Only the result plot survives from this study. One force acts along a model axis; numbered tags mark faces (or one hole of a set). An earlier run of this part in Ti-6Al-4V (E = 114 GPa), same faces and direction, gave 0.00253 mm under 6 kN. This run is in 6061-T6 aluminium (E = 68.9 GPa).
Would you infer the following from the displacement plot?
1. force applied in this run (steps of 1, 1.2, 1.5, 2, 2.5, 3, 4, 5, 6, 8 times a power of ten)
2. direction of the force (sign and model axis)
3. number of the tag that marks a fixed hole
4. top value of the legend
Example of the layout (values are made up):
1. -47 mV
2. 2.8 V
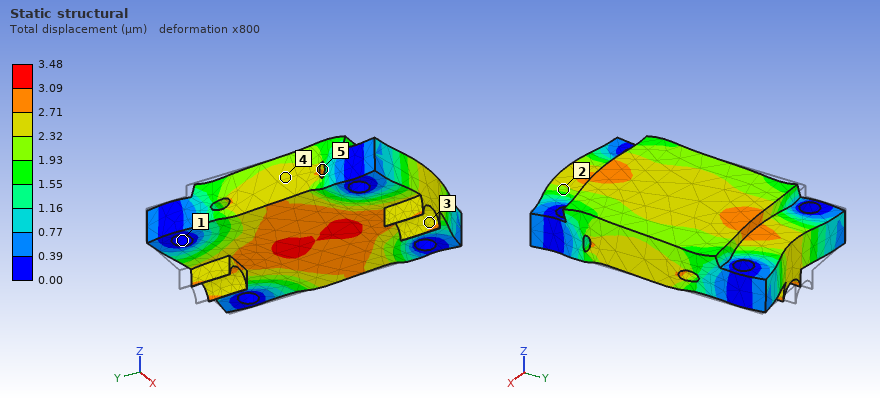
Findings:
1. 5 kN
2. -Y
3. 1
4. 3.48 µm
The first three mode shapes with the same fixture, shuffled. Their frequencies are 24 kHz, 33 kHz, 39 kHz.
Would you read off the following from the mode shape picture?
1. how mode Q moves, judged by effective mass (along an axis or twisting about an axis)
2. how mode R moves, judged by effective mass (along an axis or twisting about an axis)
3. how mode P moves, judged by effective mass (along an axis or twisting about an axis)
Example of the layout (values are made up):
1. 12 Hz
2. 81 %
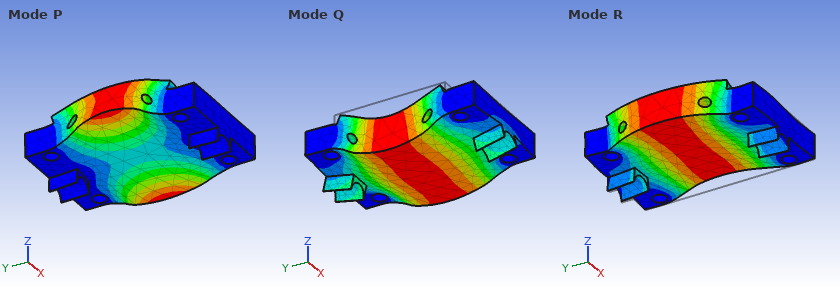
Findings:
1. along Z
2. along X
3. twisting about Y
